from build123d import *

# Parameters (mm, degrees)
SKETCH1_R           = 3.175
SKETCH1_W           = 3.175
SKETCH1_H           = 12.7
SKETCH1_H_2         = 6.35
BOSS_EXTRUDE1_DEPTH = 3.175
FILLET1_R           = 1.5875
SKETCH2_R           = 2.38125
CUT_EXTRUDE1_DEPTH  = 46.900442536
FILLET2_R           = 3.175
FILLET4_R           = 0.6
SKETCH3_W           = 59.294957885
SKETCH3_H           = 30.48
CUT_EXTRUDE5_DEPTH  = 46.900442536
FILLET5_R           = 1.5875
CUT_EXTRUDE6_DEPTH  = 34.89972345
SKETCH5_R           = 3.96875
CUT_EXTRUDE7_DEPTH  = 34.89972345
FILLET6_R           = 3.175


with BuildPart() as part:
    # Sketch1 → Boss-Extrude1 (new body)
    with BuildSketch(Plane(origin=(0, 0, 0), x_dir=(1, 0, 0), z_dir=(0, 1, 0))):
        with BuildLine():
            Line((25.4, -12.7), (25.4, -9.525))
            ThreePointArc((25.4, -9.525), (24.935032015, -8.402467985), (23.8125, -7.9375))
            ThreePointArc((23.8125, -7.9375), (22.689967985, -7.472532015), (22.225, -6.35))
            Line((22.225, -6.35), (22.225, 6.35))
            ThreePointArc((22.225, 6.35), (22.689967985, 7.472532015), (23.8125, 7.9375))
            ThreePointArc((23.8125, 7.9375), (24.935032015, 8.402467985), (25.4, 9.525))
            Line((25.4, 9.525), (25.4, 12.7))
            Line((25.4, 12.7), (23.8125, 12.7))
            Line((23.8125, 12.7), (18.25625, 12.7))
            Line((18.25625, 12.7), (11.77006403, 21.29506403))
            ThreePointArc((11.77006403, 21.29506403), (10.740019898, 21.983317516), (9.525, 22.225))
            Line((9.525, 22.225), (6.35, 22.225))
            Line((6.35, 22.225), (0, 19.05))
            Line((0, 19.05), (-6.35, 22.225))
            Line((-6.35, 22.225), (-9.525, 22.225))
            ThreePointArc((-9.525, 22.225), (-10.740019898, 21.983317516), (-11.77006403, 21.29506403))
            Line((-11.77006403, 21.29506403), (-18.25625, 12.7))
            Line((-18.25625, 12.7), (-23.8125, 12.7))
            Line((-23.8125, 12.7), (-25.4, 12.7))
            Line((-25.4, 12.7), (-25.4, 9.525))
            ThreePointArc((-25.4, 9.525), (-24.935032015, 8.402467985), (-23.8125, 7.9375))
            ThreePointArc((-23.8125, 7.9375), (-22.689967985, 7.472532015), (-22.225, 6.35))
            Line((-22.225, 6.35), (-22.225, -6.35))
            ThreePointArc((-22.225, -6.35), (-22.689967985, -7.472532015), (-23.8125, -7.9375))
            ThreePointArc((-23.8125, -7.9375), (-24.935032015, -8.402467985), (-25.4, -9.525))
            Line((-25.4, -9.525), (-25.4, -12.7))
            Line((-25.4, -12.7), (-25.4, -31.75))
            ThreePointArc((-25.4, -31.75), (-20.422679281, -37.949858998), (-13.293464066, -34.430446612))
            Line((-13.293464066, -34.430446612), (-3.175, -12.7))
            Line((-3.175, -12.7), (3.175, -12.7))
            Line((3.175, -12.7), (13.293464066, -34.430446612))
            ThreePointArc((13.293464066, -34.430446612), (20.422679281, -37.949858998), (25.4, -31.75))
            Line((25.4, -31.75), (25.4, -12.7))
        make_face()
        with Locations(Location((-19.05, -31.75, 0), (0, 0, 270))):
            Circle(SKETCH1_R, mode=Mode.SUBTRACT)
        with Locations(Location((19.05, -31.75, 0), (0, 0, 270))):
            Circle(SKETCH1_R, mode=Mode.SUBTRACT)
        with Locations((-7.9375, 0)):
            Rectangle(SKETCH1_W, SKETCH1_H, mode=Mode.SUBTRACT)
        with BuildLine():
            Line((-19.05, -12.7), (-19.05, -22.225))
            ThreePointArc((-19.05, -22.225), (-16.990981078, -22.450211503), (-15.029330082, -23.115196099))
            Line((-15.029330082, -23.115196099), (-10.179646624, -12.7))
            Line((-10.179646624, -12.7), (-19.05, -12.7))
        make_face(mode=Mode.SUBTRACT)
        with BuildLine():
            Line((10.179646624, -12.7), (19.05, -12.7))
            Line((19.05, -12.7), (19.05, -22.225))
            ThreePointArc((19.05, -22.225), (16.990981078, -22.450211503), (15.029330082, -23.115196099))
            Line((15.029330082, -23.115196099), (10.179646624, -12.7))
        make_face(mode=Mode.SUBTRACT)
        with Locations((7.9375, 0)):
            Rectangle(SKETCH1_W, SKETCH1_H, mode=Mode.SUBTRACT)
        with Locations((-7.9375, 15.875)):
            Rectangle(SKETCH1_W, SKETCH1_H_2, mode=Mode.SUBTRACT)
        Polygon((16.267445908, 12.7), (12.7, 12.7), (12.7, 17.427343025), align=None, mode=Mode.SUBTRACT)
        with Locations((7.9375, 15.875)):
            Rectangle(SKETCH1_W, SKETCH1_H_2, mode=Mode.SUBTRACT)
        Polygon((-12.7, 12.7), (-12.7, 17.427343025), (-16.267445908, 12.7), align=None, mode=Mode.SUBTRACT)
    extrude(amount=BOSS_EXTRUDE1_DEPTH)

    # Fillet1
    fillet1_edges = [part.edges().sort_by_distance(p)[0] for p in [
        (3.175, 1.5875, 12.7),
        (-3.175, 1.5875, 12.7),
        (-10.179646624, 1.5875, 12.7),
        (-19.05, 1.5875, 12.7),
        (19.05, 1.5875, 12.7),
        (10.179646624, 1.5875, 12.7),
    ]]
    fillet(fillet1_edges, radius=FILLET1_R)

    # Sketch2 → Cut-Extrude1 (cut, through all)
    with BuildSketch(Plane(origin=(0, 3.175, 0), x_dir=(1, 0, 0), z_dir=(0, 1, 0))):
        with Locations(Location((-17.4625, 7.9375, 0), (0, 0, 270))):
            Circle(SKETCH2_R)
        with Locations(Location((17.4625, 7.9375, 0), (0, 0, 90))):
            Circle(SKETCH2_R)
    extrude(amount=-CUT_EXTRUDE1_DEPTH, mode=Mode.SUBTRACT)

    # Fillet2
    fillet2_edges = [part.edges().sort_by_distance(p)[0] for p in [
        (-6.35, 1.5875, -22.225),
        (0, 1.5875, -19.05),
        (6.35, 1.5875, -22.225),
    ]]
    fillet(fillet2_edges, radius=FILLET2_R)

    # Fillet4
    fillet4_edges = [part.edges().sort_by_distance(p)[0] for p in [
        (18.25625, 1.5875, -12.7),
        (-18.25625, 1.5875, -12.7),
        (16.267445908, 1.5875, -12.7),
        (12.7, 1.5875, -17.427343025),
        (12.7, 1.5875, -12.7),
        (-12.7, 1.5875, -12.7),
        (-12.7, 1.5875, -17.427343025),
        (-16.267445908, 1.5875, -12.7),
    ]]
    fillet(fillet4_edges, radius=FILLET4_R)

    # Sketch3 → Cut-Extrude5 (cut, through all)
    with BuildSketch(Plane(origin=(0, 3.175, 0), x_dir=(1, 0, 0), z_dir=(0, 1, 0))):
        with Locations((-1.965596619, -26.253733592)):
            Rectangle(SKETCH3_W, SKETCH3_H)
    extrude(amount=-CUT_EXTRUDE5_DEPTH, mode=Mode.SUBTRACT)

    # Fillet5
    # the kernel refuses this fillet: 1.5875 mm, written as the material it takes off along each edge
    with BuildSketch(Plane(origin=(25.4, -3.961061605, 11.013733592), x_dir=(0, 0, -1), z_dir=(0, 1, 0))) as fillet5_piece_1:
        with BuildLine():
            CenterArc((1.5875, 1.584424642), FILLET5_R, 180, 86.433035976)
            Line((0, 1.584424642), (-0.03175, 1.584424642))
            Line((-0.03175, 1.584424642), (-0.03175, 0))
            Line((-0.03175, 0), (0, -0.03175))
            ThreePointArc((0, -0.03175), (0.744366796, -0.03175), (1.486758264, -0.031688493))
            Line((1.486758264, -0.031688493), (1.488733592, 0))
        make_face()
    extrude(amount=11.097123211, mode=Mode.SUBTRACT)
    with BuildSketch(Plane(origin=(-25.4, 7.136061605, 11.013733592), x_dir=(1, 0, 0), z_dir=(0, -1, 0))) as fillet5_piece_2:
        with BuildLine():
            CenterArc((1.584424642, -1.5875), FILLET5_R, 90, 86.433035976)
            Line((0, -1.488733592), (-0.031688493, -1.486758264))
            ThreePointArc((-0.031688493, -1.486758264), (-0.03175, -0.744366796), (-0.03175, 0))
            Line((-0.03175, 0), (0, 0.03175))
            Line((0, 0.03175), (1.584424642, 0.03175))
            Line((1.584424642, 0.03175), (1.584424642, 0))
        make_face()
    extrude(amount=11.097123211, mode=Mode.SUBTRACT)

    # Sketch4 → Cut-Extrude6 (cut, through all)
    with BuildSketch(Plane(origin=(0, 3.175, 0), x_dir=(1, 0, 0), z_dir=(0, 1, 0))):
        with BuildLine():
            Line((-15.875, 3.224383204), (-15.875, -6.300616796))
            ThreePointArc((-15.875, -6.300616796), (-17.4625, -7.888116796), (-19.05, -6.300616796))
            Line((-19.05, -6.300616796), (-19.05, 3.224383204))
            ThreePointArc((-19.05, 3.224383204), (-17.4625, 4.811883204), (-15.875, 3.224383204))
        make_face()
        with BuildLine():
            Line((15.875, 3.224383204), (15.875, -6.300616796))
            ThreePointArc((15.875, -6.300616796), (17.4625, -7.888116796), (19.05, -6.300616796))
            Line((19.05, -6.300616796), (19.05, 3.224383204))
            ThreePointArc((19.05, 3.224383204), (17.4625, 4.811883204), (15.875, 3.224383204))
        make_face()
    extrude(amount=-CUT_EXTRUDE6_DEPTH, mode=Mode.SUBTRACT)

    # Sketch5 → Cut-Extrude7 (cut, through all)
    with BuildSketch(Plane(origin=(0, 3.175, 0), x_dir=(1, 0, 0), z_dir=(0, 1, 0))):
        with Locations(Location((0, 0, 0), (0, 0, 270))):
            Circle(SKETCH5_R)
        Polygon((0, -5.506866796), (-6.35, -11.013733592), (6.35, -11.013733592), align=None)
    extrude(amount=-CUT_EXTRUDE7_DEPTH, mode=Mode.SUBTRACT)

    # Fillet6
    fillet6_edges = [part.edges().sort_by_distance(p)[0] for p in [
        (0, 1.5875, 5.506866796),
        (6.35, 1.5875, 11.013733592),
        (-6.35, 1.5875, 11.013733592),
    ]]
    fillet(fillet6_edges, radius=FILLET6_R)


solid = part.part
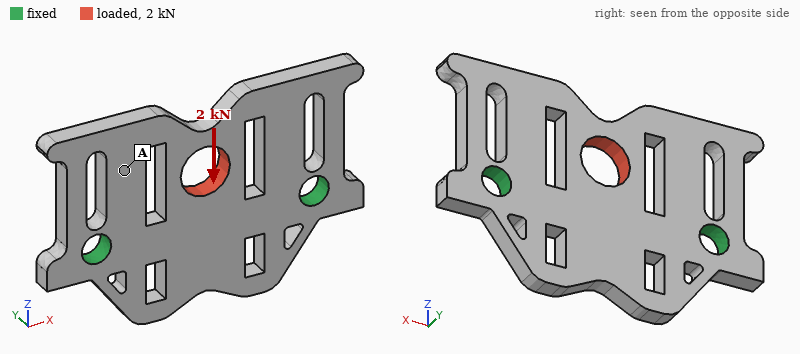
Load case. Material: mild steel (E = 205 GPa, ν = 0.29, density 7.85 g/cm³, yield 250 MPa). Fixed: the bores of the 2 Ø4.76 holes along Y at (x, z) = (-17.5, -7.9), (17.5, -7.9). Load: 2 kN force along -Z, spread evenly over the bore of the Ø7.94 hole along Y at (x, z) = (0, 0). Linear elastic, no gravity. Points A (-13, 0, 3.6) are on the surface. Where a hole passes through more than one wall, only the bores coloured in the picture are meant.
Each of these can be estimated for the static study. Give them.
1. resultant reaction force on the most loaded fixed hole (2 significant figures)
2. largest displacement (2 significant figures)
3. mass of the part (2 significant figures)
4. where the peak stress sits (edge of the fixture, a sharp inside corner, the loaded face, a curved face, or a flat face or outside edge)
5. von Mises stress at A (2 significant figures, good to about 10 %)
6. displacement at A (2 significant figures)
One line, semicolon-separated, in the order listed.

1.0 kN; 15 µm; 26 g; a curved face; 23 MPa; 3.6 µm
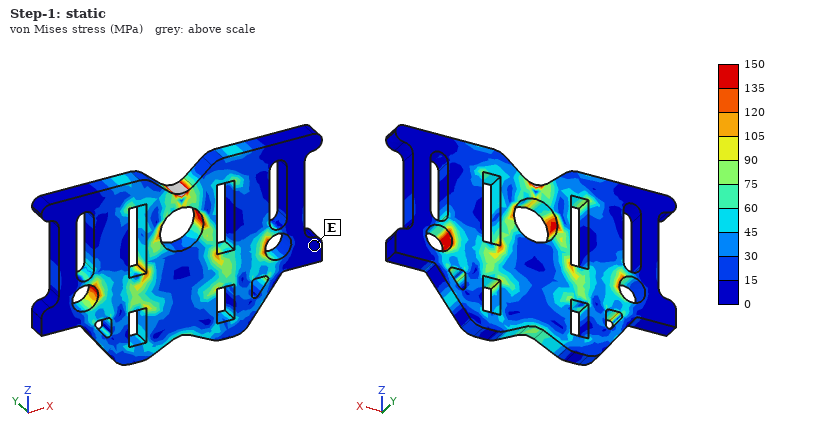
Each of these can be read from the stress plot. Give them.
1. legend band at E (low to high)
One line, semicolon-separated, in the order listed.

0 to 15 MPa
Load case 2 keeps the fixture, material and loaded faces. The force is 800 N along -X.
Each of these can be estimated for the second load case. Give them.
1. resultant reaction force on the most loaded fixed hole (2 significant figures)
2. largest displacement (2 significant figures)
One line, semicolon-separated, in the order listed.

430 N; 5.0 µm
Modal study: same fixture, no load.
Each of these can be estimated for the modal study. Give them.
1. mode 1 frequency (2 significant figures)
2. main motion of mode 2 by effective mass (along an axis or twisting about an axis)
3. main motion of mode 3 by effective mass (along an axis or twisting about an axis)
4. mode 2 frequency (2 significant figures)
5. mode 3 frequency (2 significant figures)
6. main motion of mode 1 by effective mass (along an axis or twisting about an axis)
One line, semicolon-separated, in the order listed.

5900 Hz; twisting about Z; along Y; 8000 Hz; 10 kHz; along Y
